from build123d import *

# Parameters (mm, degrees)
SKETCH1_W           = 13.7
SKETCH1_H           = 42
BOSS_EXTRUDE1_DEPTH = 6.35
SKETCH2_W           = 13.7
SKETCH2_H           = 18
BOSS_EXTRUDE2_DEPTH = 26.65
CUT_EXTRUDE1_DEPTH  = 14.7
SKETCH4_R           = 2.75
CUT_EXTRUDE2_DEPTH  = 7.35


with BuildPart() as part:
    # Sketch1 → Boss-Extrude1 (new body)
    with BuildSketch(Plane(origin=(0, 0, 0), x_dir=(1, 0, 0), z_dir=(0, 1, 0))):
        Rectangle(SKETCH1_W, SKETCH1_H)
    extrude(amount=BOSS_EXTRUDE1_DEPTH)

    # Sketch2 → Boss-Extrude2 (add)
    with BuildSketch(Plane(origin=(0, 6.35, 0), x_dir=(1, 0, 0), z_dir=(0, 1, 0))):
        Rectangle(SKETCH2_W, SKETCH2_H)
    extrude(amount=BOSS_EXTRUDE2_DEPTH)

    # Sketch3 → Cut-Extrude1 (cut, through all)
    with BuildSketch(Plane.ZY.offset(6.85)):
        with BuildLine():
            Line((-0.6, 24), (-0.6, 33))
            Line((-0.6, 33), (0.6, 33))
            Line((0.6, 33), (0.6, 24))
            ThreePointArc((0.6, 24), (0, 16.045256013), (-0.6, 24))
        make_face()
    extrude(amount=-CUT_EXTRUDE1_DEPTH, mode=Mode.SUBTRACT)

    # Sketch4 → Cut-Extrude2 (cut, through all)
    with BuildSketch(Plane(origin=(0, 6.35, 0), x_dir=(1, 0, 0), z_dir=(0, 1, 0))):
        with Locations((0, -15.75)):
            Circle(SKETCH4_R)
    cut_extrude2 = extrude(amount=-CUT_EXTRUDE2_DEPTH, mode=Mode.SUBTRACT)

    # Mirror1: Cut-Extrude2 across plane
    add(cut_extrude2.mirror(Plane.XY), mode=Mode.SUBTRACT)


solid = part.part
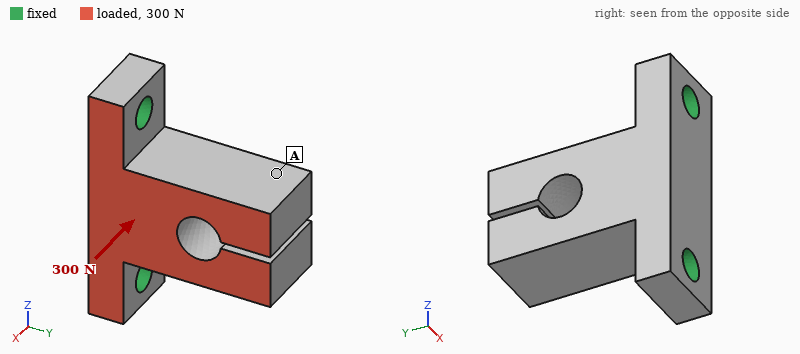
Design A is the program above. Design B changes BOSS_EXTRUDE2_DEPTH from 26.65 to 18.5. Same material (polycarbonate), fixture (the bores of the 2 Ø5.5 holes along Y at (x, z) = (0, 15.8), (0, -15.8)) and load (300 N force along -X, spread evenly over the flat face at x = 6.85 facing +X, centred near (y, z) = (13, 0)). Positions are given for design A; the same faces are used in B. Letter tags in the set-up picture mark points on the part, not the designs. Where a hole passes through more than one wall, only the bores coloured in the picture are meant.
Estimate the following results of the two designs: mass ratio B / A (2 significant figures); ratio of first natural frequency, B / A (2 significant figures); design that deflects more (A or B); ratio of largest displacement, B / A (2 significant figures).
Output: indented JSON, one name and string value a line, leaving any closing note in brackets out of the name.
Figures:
{
  "mass ratio B / A": "0.79",
  "ratio of first natural frequency, B / A": "1.7",
  "design that deflects more": "A",
  "ratio of largest displacement, B / A": "0.45"
}
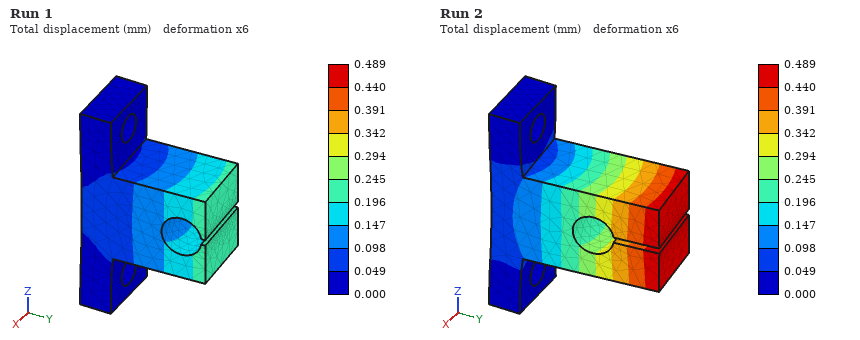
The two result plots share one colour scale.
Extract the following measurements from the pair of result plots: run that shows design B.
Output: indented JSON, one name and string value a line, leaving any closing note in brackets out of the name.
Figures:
{
  "run that shows design B": "Run 1"
}
